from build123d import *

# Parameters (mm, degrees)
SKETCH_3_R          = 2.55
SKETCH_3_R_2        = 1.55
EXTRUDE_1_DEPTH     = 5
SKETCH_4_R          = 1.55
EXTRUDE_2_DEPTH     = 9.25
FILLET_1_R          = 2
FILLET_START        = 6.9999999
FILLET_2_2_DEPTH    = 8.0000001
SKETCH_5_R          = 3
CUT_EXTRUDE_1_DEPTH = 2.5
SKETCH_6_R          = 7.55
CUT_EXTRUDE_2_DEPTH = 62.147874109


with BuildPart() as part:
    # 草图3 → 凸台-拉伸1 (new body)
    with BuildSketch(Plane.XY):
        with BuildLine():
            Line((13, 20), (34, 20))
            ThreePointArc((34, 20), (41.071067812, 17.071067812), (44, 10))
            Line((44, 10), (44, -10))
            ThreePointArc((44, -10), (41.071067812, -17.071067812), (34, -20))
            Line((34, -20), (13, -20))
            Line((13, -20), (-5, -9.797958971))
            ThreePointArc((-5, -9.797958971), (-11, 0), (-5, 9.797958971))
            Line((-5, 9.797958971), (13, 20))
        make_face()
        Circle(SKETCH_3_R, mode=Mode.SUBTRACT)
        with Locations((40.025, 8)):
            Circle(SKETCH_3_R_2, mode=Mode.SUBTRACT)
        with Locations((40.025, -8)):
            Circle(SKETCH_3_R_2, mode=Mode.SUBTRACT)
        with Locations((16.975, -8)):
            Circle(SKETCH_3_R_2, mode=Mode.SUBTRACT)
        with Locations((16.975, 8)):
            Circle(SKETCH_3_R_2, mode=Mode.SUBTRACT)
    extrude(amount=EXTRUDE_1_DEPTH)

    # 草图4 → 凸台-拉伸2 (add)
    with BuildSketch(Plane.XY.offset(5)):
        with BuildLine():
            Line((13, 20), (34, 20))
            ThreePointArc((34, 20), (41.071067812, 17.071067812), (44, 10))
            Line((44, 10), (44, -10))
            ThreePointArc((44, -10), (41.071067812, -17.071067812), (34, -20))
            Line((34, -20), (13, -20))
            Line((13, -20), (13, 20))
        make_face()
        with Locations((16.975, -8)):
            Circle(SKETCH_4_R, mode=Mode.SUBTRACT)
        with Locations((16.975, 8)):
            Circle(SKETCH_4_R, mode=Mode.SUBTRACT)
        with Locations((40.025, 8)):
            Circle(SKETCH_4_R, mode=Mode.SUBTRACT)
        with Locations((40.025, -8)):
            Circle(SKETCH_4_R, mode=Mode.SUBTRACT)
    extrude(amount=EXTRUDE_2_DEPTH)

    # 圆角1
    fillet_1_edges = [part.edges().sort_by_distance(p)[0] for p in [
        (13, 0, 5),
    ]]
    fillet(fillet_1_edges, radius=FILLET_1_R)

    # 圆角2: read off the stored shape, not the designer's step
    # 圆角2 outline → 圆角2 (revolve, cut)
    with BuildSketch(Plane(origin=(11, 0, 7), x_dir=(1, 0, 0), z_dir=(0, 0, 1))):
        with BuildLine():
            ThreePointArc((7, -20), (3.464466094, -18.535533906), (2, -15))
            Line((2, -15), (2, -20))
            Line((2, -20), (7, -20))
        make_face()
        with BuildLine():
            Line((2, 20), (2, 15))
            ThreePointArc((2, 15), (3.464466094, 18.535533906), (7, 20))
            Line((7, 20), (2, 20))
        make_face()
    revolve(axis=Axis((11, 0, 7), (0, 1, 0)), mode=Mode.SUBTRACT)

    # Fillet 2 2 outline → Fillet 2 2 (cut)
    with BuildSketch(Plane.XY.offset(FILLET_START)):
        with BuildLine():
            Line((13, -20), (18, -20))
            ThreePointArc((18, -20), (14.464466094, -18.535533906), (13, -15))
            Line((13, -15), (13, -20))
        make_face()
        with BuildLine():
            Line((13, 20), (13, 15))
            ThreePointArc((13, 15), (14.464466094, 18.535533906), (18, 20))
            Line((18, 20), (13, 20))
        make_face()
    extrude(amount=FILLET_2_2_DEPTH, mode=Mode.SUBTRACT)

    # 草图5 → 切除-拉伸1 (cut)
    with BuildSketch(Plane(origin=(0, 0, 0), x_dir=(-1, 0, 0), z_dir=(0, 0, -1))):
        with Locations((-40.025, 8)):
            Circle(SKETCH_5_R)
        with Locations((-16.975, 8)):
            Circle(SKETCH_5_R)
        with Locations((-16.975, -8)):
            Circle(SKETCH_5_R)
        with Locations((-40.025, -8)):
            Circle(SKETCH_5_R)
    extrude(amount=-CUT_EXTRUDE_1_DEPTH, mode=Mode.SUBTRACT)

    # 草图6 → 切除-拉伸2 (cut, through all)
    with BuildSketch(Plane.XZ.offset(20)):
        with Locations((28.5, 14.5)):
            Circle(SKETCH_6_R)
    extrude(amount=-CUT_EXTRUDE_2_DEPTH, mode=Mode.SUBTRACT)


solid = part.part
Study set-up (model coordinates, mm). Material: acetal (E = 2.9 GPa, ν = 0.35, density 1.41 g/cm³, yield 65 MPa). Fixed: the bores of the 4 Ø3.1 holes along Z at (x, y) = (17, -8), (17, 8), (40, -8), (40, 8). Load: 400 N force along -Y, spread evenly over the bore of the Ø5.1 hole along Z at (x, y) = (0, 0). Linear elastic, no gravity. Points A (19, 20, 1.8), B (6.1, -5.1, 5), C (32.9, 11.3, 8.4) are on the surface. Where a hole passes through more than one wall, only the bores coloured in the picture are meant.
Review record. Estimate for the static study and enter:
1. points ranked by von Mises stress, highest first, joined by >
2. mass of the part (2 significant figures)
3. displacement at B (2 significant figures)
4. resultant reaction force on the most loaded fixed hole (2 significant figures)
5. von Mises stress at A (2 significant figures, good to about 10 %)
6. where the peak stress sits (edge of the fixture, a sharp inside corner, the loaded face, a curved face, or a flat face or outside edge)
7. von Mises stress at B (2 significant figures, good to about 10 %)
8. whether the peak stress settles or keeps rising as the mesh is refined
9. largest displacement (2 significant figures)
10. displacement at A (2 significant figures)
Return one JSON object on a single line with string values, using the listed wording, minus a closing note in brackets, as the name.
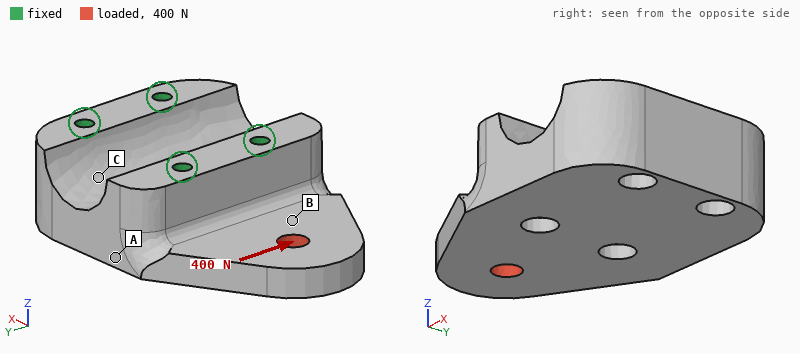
{"points ranked by von Mises stress, highest first, joined by >": "B > A > C", "mass of the part": "22 g", "displacement at B": "37 µm", "resultant reaction force on the most loaded fixed hole": "310 N", "von Mises stress at A": "3.7 MPa", "where the peak stress sits": "edge of the fixture", "von Mises stress at B": "5.3 MPa", "whether the peak stress settles or keeps rising as the mesh is refined": "keeps rising", "largest displacement": "83 µm", "displacement at A": "19 µm"}
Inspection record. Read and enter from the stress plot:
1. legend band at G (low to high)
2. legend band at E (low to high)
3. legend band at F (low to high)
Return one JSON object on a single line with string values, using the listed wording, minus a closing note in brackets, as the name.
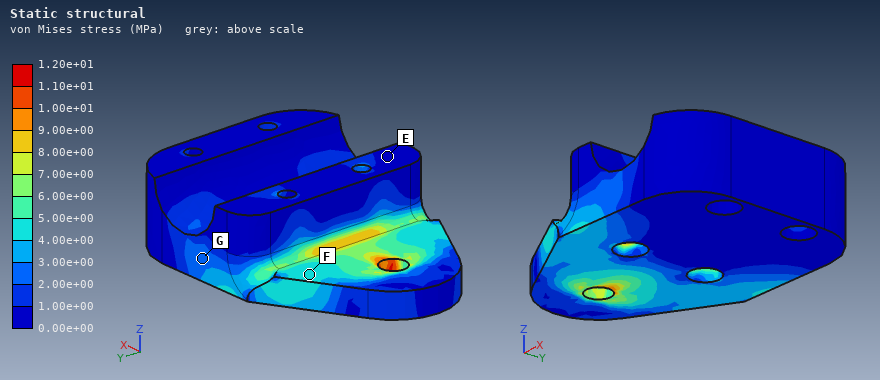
{"legend band at G": "2.00e+00 to 3.00e+00 MPa", "legend band at E": "0.00e+00 to 1.00e+00 MPa", "legend band at F": "4.00e+00 to 5.00e+00 MPa"}
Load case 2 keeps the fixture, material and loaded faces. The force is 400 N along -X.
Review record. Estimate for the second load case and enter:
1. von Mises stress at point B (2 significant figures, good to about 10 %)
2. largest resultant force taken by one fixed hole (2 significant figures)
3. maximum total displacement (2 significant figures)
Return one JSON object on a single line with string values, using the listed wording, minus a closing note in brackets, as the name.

{"von Mises stress at point B": "3.7 MPa", "largest resultant force taken by one fixed hole": "160 N", "maximum total displacement": "57 µm"}
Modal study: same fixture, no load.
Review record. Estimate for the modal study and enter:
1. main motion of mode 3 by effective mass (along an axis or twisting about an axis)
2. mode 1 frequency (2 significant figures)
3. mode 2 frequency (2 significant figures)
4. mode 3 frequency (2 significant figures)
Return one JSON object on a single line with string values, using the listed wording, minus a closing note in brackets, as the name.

{"main motion of mode 3 by effective mass": "along Y", "mode 1 frequency": "2300 Hz", "mode 2 frequency": "5600 Hz", "mode 3 frequency": "6900 Hz"}
